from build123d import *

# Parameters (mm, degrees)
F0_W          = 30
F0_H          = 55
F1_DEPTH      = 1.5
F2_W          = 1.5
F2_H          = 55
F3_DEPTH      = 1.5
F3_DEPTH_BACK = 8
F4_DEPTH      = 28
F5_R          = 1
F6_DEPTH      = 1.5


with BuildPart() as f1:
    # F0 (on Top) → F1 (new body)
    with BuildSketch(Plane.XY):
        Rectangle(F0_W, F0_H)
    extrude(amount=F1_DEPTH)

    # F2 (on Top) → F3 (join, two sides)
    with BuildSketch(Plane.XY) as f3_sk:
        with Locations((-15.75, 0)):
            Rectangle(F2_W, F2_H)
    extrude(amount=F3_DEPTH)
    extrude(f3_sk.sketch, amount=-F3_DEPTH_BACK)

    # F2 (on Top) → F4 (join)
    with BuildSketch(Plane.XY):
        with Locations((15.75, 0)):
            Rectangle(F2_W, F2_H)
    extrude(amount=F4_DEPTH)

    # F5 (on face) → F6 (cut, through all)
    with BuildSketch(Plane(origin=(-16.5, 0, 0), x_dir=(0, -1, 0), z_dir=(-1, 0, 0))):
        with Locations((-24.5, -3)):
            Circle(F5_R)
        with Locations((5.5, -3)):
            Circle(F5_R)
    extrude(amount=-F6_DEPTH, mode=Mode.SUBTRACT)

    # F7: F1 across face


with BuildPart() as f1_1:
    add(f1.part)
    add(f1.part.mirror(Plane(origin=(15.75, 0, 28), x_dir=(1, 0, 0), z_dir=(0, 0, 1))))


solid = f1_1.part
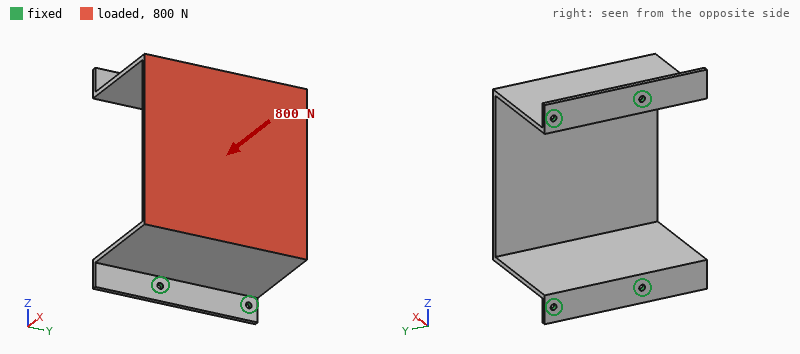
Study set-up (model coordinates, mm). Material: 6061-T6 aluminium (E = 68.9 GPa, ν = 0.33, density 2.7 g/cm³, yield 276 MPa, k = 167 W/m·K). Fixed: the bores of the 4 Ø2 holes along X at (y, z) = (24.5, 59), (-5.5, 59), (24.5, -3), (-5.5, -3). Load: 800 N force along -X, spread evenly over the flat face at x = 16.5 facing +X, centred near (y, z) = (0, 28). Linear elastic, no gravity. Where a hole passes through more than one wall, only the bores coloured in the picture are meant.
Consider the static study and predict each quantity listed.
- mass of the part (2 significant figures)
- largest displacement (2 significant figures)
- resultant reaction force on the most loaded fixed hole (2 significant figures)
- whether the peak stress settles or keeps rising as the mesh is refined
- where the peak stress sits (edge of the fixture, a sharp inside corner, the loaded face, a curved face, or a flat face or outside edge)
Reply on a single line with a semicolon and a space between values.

30 g; 0.62 mm; 330 N; keeps rising; edge of the fixture
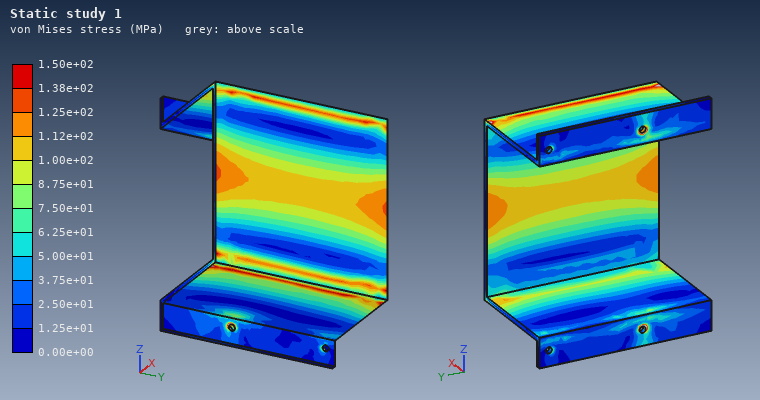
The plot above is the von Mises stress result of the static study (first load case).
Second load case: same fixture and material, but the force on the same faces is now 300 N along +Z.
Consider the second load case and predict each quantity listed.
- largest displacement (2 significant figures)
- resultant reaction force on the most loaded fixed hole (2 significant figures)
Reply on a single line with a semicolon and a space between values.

0.83 mm; 120 N
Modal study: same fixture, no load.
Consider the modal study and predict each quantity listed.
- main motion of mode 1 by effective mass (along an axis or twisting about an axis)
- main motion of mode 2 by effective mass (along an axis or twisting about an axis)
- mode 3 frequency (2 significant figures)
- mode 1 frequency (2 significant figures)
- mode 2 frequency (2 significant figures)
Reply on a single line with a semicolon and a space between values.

along Z; along X; 2500 Hz; 740 Hz; 1900 Hz
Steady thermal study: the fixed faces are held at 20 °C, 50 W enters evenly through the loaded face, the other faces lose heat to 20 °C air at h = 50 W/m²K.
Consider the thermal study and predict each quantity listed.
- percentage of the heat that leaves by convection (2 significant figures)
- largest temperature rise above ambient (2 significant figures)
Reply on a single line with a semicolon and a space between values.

44 %; 69 K
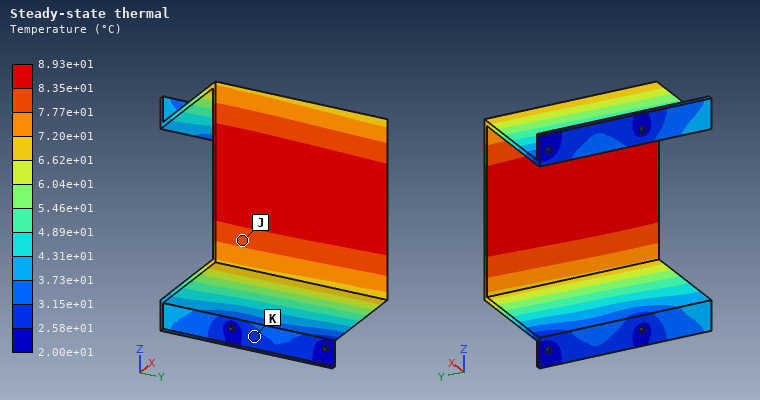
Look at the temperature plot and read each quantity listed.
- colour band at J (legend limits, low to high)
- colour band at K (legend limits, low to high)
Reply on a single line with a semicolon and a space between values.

7.77e+01 to 8.35e+01 °C; 2.58e+01 to 3.15e+01 °C
